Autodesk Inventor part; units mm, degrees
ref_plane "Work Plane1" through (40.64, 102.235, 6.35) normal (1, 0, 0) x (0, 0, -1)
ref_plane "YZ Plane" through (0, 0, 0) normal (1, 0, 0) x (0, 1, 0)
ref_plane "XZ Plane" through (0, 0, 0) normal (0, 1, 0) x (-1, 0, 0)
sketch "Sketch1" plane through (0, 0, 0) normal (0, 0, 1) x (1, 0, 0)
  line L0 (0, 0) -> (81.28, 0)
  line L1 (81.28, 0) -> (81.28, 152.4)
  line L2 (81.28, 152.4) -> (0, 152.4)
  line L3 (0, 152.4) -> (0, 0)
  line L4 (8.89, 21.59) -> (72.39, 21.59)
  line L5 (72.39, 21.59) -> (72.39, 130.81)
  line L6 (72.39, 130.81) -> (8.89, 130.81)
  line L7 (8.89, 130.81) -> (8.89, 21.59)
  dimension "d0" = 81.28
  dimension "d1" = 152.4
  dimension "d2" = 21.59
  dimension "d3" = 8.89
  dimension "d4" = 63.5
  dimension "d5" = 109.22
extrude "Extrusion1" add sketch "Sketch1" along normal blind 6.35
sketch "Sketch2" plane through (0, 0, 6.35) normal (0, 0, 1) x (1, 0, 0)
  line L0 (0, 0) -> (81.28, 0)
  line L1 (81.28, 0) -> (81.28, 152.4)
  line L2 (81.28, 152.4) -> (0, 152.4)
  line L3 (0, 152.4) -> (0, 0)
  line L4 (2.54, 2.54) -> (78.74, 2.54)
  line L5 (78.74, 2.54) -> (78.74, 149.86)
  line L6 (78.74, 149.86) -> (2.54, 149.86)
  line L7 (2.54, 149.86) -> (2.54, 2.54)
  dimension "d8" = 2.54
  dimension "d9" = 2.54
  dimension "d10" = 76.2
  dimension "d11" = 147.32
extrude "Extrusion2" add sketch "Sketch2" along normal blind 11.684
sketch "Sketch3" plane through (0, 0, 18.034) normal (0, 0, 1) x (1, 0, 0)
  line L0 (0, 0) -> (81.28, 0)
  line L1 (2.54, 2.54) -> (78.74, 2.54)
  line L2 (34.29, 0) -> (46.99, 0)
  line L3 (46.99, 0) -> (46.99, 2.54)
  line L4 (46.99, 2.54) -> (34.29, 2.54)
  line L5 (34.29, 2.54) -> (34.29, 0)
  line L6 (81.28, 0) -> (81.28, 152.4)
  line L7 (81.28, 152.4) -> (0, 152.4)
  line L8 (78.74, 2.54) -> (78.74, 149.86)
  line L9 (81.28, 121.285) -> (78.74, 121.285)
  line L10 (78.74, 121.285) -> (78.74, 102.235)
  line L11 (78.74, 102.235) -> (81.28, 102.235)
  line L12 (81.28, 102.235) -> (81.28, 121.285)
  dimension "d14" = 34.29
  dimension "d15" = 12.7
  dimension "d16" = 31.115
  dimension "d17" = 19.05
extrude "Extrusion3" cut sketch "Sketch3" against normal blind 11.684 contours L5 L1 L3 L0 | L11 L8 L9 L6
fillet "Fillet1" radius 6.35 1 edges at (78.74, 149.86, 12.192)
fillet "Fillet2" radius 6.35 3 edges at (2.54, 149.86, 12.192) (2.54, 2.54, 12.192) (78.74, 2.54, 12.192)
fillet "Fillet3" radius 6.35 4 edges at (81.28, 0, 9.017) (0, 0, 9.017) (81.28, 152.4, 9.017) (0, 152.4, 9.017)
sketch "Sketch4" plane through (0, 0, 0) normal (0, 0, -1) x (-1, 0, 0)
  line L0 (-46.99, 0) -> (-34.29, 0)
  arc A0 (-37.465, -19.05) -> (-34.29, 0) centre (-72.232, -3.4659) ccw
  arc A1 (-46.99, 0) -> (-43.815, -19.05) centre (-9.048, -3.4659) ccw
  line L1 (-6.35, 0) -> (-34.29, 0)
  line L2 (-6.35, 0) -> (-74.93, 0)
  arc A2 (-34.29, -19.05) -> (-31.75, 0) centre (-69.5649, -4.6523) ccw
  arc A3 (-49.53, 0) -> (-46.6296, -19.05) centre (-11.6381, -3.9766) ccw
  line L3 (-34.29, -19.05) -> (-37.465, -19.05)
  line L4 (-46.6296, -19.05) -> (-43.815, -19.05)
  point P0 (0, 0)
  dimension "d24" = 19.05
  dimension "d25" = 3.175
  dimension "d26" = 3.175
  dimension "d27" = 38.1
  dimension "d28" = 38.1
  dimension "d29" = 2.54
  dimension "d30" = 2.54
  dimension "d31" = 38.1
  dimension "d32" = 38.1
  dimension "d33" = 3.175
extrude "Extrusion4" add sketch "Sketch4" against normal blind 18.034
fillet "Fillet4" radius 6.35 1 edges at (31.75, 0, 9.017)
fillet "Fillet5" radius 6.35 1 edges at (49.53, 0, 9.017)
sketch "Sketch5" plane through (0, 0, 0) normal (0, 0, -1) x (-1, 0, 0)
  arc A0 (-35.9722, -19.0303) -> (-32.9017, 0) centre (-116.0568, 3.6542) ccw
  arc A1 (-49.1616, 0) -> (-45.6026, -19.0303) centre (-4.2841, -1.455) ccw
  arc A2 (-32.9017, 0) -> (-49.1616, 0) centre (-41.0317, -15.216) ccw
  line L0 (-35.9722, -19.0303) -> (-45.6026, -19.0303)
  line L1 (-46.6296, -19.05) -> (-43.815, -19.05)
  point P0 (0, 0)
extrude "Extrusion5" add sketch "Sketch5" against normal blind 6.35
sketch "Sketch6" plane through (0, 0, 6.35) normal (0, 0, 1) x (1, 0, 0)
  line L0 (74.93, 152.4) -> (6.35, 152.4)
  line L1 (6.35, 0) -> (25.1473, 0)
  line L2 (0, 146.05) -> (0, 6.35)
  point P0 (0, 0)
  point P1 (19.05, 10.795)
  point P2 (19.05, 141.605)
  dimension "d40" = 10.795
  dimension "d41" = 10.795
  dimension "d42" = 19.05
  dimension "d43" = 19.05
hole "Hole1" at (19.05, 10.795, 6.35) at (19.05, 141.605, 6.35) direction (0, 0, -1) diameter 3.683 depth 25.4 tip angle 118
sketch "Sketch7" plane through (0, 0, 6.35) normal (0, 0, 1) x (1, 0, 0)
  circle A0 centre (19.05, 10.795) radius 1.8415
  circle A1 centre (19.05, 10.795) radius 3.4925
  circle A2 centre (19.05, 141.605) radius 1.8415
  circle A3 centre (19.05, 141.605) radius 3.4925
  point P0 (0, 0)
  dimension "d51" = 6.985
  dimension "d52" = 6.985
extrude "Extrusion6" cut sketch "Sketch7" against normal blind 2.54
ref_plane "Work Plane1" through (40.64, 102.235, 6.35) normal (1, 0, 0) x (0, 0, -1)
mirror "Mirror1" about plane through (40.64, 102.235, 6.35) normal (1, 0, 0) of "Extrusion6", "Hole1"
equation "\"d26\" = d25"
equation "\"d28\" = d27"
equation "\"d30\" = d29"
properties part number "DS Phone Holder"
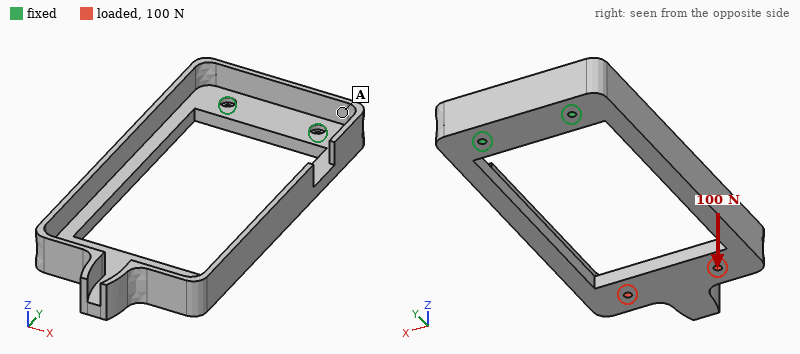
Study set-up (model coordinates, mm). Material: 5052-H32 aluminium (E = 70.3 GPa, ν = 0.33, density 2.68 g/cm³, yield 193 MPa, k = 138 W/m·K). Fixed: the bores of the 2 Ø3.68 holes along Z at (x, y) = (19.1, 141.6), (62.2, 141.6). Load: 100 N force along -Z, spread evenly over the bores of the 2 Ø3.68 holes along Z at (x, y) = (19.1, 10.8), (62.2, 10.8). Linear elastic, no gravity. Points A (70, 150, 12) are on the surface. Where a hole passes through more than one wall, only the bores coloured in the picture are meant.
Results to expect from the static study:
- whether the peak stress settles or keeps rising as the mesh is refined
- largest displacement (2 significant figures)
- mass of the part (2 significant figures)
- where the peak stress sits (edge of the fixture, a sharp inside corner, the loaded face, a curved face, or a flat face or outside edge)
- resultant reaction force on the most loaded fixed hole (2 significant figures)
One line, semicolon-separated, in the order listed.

keeps rising; 1.4 mm; 130 g; edge of the fixture; 110 N
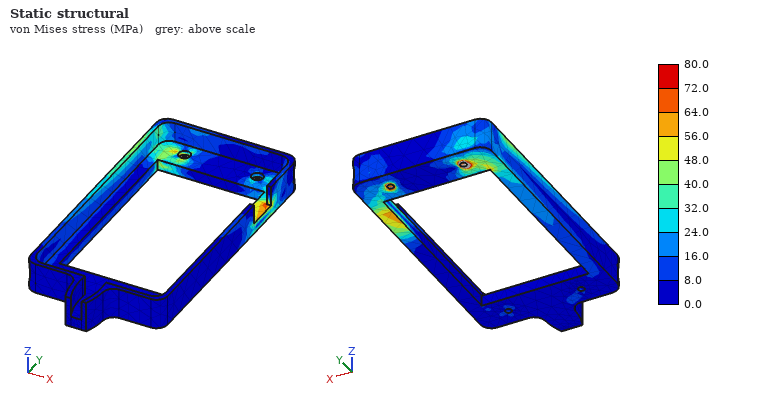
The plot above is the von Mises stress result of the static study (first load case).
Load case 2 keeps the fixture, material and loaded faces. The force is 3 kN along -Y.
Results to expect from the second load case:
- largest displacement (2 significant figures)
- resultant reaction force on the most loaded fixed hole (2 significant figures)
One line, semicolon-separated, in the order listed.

0.66 mm; 1.5 kN
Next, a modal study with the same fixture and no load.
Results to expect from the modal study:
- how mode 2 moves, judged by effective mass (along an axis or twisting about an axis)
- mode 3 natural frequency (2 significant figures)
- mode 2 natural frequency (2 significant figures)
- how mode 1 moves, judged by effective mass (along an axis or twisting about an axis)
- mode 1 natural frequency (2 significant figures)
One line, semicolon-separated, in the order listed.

along X; 560 Hz; 370 Hz; along Z; 190 Hz
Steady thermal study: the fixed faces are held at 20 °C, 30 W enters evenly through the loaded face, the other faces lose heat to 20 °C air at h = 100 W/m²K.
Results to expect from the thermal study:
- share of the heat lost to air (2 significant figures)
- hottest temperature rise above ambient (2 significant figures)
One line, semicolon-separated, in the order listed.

96 %; 31 K
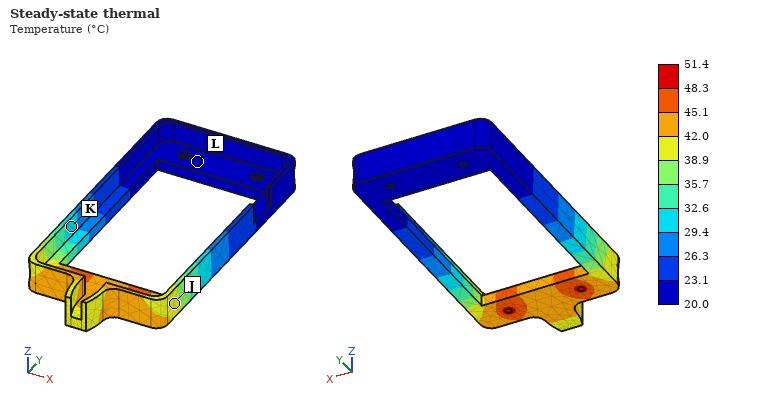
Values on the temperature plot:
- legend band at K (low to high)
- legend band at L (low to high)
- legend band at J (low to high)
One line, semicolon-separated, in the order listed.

29.4 to 32.6 °C; 20.0 to 23.1 °C; 38.9 to 42.0 °C
